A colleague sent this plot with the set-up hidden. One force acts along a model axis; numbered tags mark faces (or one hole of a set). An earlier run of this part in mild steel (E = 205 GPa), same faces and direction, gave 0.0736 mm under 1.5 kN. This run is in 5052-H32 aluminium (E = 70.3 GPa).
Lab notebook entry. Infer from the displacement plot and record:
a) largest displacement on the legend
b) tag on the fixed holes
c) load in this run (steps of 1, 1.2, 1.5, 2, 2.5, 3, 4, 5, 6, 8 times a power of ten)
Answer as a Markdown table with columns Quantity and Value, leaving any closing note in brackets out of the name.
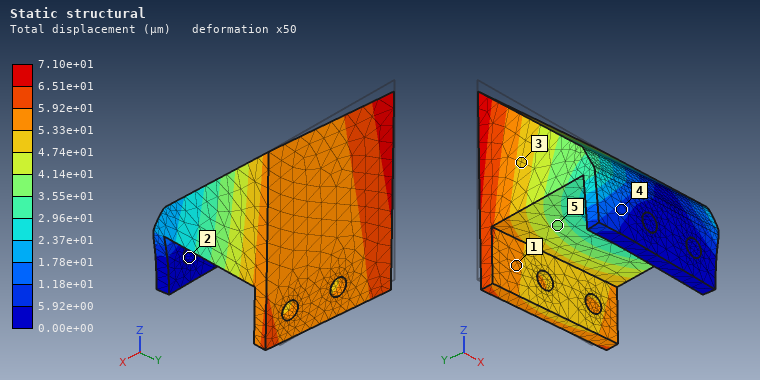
| Quantity | Value |
|---|---|
| largest displacement on the legend | 7.10e+01 µm |
| tag on the fixed holes | 2 |
| load in this run | 500 N |
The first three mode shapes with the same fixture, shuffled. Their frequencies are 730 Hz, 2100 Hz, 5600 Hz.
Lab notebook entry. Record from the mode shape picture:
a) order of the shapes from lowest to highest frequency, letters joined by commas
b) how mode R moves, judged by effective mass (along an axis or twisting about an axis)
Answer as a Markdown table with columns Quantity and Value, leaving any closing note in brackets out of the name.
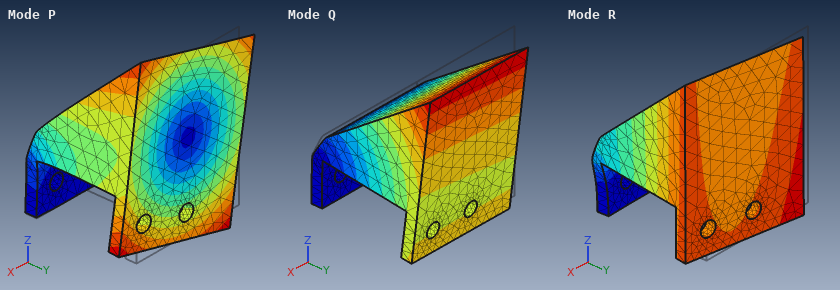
| Quantity | Value |
|---|---|
| order of the shapes from lowest to highest frequency, letters joined by commas | Q, R, P |
| how mode R moves, judged by effective mass | along X |
